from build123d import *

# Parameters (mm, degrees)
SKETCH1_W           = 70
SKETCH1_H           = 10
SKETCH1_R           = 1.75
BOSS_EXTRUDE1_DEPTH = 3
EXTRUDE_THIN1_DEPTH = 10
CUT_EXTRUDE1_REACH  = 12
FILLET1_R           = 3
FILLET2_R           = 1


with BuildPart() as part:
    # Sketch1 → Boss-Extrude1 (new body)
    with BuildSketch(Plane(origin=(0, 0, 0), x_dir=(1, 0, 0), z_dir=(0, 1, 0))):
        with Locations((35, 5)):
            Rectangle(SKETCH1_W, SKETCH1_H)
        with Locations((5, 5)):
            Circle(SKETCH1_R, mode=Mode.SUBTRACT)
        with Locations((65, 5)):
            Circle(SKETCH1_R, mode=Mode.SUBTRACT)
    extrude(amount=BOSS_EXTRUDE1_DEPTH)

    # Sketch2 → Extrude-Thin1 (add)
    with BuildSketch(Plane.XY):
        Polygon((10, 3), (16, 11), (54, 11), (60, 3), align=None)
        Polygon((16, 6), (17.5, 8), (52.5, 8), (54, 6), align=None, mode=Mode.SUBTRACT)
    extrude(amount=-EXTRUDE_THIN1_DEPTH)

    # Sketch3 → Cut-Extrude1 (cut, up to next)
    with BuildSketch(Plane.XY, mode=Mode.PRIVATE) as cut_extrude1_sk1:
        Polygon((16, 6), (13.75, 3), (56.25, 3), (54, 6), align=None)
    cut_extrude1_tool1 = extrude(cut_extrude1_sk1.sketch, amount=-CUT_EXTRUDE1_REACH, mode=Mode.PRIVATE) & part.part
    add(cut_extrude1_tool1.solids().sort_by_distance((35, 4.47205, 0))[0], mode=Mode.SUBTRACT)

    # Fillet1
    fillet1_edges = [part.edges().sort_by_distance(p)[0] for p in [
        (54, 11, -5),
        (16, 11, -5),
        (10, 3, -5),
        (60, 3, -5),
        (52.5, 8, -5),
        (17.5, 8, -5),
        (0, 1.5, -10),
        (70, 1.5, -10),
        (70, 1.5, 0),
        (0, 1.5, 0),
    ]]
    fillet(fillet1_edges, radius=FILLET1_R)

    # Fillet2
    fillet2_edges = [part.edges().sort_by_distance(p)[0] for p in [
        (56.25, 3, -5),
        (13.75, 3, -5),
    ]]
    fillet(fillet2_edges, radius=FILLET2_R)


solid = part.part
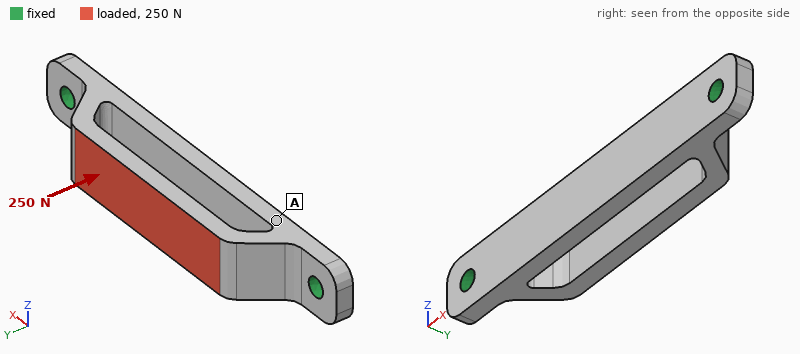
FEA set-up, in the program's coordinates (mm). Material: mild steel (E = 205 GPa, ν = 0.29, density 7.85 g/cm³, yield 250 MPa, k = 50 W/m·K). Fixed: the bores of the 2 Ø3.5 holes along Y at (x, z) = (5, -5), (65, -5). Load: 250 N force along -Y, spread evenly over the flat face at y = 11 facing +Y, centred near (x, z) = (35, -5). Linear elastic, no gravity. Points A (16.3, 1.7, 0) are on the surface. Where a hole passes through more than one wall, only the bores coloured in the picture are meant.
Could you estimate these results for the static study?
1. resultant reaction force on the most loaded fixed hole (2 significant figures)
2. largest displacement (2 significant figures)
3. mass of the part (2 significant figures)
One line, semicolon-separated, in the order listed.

210 N; 13 µm; 28 g
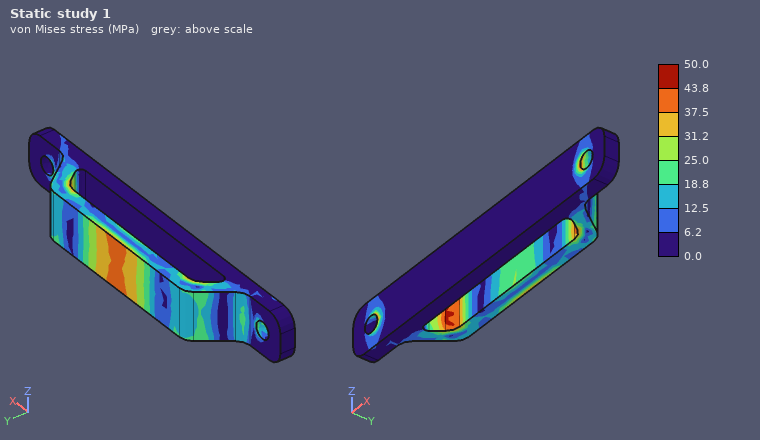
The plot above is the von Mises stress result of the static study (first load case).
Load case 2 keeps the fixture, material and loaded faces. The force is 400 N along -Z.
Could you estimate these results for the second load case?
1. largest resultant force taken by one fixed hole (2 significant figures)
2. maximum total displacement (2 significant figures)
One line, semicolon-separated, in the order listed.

200 N; 23 µm
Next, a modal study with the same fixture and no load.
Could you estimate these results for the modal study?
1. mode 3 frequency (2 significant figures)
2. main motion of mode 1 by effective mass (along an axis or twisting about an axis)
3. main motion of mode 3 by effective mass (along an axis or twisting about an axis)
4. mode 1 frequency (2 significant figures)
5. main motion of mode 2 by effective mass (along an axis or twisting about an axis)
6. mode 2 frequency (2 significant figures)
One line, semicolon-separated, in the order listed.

8900 Hz; along Y; along Y; 6800 Hz; along Z; 7400 Hz
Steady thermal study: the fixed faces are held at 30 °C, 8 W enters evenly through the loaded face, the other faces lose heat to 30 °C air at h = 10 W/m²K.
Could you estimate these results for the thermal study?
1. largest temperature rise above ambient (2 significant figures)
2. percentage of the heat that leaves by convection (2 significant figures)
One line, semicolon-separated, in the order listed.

58 K; 7.4 %
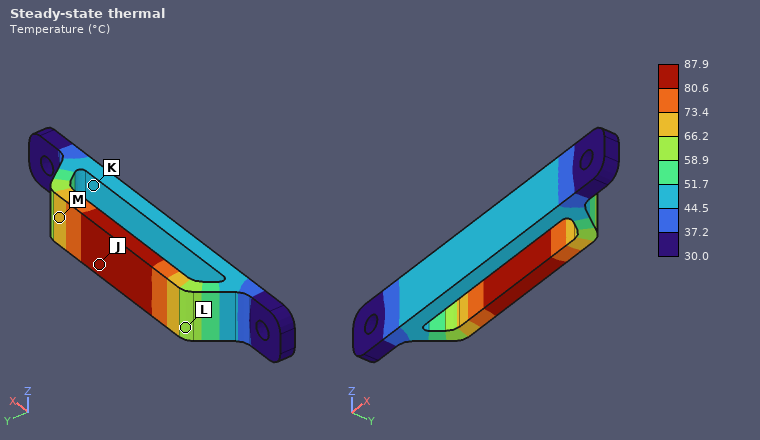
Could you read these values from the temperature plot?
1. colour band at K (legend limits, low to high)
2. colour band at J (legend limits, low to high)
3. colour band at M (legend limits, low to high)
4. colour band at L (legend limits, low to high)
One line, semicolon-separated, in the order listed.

44.5 to 51.7 °C; 80.6 to 87.9 °C; 66.2 to 73.4 °C; 58.9 to 66.2 °C
